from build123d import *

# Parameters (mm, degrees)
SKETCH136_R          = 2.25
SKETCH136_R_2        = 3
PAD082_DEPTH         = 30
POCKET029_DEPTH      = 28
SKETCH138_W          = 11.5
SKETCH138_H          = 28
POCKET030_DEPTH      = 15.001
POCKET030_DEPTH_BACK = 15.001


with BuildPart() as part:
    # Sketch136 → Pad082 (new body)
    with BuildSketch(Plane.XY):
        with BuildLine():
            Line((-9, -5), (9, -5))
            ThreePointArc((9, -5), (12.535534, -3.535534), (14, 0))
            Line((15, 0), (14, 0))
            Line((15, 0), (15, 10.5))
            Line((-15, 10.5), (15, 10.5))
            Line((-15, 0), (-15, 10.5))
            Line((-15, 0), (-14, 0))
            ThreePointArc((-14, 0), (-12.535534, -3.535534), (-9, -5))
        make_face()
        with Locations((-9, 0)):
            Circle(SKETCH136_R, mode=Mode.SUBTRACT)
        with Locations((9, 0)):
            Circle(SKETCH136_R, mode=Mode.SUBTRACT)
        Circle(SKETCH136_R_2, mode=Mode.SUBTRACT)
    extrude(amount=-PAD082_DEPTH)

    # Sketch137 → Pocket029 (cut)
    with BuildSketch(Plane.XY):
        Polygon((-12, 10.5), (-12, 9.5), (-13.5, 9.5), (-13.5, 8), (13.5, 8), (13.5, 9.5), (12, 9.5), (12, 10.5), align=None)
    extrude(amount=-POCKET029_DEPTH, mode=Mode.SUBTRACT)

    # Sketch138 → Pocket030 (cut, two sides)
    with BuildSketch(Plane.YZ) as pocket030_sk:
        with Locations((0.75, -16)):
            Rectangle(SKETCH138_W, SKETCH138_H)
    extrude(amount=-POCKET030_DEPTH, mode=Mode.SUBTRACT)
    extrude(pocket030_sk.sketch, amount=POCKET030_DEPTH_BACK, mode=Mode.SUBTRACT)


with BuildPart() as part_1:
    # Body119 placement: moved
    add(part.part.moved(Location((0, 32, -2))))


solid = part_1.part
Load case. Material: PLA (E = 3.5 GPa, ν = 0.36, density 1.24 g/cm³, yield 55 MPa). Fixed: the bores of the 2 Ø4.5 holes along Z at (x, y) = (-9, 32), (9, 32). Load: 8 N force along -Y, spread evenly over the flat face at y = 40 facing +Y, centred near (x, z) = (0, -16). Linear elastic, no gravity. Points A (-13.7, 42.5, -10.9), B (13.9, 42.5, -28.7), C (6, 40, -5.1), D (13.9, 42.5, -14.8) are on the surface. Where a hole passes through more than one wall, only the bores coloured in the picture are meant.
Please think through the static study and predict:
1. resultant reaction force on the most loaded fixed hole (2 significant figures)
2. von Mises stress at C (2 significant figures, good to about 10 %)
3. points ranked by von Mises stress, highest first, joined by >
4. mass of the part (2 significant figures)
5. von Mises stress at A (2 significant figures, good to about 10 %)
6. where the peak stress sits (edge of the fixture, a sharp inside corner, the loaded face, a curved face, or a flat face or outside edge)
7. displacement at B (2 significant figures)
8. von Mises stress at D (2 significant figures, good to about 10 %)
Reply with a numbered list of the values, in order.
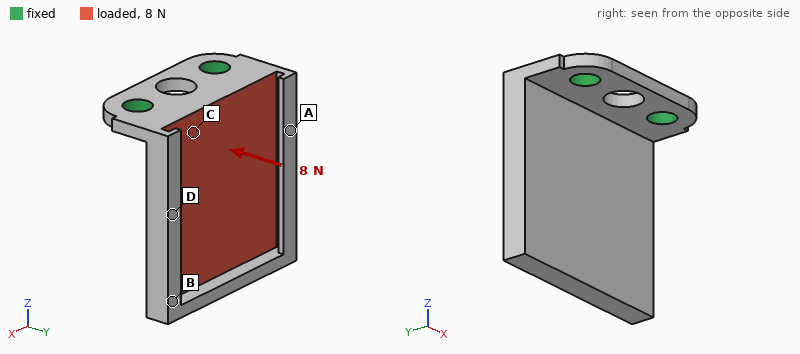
1. 4.3 N
2. 4.5 MPa
3. C > A > D > B
4. 2.9 g
5. 2.4 MPa
6. a flat face or outside edge
7. 0.44 mm
8. 1.7 MPa
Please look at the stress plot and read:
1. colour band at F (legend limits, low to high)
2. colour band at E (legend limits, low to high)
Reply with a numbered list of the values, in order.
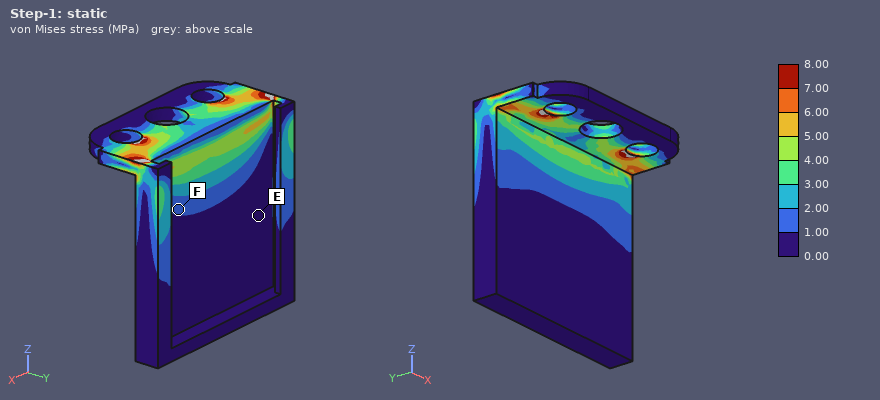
1. 1.00 to 2.00 MPa
2. 0.00 to 1.00 MPa
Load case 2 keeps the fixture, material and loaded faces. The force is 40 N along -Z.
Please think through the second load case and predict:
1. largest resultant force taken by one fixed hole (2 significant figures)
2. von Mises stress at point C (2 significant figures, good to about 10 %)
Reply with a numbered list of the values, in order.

1. 20 N
2. 2.0 MPa
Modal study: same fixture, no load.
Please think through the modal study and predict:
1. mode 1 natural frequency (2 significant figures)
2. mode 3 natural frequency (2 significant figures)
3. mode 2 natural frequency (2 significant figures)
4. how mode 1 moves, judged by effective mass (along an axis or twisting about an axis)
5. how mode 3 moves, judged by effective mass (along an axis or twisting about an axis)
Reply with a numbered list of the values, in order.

1. 460 Hz
2. 1800 Hz
3. 1000 Hz
4. along Y
5. along X
